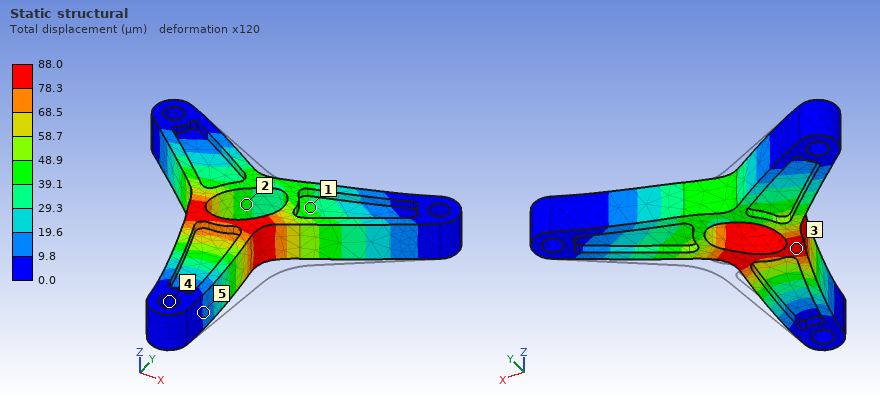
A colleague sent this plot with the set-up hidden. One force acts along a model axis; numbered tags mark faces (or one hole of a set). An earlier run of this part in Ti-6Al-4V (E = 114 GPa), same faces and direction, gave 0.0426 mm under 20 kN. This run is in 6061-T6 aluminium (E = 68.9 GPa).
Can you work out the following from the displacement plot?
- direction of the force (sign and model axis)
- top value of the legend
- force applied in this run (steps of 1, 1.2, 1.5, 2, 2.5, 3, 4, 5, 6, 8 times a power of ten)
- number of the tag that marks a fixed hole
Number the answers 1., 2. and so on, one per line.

1. -X
2. 88.0 µm
3. 25 kN
4. 4
